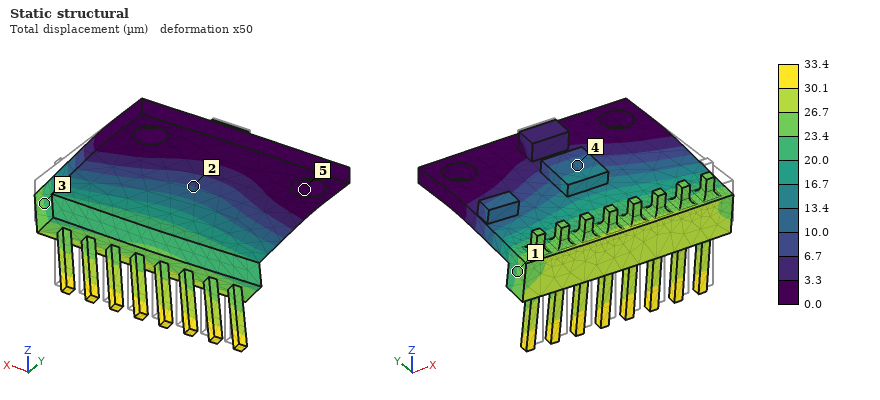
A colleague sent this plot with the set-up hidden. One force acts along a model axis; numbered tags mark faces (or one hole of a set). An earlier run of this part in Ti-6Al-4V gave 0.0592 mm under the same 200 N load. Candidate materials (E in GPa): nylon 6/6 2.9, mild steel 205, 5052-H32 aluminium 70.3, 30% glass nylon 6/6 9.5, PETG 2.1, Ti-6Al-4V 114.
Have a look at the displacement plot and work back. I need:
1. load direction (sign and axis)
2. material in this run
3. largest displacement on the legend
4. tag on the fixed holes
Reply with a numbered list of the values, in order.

1. -Z
2. mild steel
3. 33.4 µm
4. 5
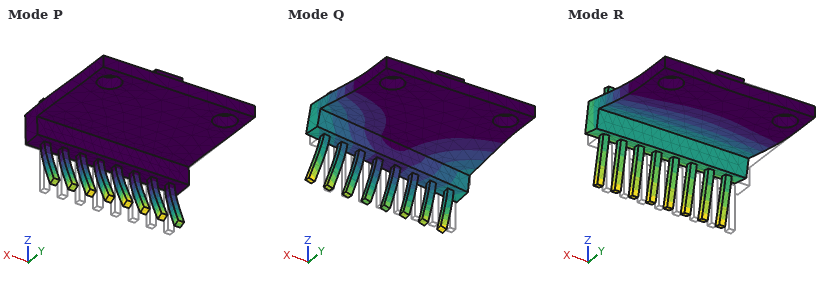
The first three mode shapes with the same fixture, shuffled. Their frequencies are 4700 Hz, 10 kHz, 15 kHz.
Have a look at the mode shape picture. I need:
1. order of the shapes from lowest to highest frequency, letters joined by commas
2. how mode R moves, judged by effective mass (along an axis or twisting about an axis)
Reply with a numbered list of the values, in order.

1. R, Q, P
2. along Z
